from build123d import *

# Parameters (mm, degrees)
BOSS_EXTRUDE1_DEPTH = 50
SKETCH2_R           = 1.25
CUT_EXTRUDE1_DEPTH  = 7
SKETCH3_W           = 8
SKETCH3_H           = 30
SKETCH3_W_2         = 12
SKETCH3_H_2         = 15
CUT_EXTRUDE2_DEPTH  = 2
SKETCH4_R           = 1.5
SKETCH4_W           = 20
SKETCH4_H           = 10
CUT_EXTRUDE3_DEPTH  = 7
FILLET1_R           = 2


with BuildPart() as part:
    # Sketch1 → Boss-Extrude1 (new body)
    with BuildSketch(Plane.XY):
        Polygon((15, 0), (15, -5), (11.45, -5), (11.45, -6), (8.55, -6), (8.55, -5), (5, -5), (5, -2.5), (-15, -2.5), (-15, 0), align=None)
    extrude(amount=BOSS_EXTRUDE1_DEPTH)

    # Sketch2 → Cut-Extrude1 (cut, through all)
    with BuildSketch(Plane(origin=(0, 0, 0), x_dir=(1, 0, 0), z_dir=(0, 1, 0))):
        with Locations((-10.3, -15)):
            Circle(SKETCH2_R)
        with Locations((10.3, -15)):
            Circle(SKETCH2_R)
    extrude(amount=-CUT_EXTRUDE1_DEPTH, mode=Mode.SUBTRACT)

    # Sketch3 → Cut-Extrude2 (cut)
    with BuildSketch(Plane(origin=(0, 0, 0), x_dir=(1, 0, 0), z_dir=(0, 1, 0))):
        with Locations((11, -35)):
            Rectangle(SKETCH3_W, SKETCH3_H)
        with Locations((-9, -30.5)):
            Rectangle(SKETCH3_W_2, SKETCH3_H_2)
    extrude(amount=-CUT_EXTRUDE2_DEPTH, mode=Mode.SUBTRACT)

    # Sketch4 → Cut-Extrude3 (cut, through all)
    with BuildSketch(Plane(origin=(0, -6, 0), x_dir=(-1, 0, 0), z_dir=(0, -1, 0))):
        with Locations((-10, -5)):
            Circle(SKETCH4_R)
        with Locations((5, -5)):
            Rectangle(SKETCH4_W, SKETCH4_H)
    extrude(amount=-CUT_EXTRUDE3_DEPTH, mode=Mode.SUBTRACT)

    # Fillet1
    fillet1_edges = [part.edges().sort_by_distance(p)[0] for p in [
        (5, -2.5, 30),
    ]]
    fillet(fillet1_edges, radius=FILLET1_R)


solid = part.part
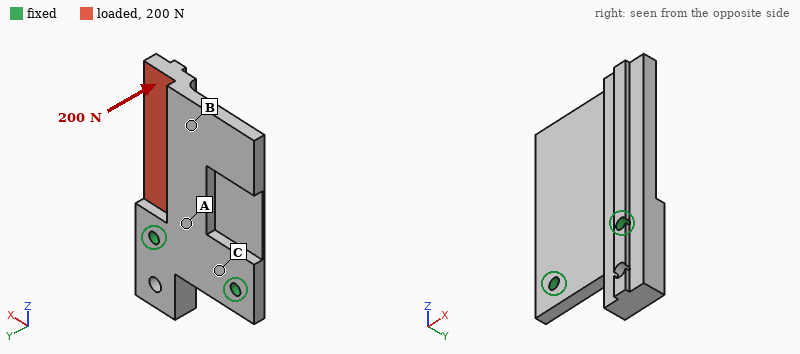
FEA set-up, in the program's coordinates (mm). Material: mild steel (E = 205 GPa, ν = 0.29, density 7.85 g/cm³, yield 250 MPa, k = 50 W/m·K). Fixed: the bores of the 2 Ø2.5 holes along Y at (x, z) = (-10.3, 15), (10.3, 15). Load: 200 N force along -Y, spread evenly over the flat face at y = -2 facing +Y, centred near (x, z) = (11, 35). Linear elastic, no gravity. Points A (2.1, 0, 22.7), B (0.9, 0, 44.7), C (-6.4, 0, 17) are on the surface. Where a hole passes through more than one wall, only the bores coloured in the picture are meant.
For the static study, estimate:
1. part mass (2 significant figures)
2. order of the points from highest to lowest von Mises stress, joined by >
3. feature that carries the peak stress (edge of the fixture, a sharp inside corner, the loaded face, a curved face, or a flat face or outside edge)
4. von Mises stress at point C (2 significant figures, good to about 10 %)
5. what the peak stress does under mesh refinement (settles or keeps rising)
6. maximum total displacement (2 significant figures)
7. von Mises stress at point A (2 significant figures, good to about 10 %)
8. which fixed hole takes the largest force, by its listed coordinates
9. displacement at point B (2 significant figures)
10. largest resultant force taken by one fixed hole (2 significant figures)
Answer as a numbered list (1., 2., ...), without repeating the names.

1. 29 g
2. A > C > B
3. edge of the fixture
4. 23 MPa
5. keeps rising
6. 68 µm
7. 45 MPa
8. (10.3, 15)
9. 44 µm
10. 220 N
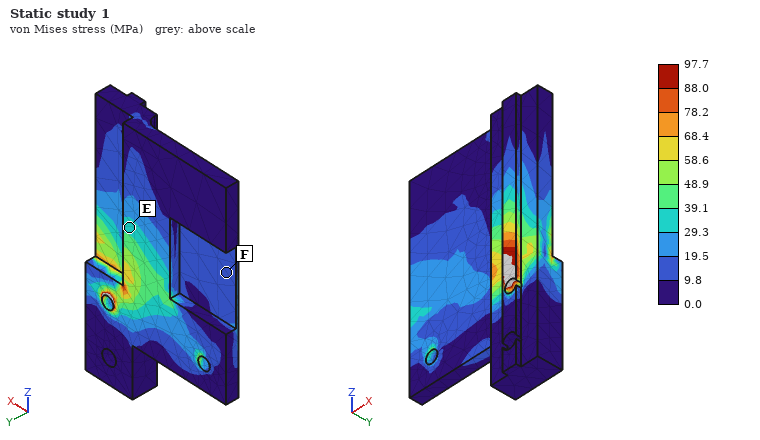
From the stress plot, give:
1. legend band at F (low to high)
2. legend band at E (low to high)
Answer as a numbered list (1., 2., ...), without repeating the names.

1. 9.8 to 19.5 MPa
2. 29.3 to 39.1 MPa
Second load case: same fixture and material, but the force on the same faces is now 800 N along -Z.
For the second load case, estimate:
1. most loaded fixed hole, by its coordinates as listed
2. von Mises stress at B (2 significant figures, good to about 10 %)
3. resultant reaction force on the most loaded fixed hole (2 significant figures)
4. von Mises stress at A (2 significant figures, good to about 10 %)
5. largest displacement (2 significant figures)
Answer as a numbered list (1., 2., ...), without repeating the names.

1. (10.3, 15)
2. 7.0 MPa
3. 820 N
4. 20 MPa
5. 29 µm
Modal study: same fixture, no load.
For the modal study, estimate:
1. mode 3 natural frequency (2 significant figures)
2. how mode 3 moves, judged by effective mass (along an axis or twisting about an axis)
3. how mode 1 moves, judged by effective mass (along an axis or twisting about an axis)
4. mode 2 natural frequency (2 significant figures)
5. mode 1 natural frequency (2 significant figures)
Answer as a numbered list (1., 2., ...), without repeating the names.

1. 11 kHz
2. along X
3. along Y
4. 4600 Hz
5. 2300 Hz
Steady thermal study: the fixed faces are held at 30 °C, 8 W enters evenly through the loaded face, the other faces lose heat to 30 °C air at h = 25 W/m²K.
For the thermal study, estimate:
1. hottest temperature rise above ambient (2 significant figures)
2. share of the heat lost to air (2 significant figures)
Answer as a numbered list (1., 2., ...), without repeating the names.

1. 45 K
2. 18 %
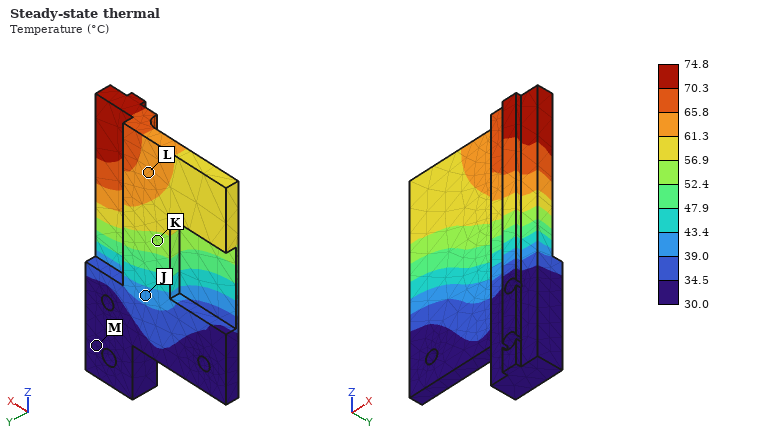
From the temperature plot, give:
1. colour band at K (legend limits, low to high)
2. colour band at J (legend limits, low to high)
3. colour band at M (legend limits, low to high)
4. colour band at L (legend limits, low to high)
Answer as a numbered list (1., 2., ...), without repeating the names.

1. 52.4 to 56.9 °C
2. 39.0 to 43.4 °C
3. 30.0 to 34.5 °C
4. 61.3 to 65.8 °C
